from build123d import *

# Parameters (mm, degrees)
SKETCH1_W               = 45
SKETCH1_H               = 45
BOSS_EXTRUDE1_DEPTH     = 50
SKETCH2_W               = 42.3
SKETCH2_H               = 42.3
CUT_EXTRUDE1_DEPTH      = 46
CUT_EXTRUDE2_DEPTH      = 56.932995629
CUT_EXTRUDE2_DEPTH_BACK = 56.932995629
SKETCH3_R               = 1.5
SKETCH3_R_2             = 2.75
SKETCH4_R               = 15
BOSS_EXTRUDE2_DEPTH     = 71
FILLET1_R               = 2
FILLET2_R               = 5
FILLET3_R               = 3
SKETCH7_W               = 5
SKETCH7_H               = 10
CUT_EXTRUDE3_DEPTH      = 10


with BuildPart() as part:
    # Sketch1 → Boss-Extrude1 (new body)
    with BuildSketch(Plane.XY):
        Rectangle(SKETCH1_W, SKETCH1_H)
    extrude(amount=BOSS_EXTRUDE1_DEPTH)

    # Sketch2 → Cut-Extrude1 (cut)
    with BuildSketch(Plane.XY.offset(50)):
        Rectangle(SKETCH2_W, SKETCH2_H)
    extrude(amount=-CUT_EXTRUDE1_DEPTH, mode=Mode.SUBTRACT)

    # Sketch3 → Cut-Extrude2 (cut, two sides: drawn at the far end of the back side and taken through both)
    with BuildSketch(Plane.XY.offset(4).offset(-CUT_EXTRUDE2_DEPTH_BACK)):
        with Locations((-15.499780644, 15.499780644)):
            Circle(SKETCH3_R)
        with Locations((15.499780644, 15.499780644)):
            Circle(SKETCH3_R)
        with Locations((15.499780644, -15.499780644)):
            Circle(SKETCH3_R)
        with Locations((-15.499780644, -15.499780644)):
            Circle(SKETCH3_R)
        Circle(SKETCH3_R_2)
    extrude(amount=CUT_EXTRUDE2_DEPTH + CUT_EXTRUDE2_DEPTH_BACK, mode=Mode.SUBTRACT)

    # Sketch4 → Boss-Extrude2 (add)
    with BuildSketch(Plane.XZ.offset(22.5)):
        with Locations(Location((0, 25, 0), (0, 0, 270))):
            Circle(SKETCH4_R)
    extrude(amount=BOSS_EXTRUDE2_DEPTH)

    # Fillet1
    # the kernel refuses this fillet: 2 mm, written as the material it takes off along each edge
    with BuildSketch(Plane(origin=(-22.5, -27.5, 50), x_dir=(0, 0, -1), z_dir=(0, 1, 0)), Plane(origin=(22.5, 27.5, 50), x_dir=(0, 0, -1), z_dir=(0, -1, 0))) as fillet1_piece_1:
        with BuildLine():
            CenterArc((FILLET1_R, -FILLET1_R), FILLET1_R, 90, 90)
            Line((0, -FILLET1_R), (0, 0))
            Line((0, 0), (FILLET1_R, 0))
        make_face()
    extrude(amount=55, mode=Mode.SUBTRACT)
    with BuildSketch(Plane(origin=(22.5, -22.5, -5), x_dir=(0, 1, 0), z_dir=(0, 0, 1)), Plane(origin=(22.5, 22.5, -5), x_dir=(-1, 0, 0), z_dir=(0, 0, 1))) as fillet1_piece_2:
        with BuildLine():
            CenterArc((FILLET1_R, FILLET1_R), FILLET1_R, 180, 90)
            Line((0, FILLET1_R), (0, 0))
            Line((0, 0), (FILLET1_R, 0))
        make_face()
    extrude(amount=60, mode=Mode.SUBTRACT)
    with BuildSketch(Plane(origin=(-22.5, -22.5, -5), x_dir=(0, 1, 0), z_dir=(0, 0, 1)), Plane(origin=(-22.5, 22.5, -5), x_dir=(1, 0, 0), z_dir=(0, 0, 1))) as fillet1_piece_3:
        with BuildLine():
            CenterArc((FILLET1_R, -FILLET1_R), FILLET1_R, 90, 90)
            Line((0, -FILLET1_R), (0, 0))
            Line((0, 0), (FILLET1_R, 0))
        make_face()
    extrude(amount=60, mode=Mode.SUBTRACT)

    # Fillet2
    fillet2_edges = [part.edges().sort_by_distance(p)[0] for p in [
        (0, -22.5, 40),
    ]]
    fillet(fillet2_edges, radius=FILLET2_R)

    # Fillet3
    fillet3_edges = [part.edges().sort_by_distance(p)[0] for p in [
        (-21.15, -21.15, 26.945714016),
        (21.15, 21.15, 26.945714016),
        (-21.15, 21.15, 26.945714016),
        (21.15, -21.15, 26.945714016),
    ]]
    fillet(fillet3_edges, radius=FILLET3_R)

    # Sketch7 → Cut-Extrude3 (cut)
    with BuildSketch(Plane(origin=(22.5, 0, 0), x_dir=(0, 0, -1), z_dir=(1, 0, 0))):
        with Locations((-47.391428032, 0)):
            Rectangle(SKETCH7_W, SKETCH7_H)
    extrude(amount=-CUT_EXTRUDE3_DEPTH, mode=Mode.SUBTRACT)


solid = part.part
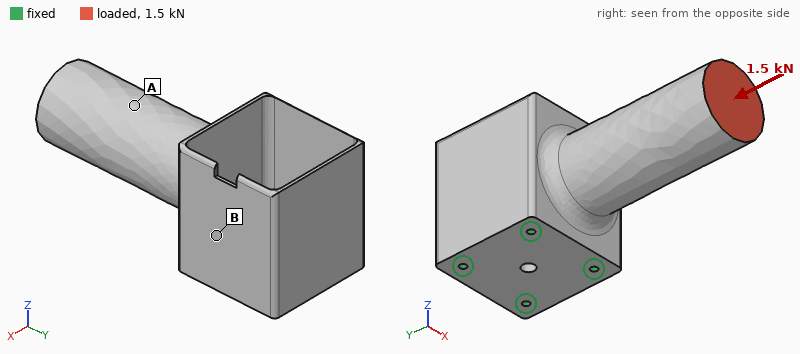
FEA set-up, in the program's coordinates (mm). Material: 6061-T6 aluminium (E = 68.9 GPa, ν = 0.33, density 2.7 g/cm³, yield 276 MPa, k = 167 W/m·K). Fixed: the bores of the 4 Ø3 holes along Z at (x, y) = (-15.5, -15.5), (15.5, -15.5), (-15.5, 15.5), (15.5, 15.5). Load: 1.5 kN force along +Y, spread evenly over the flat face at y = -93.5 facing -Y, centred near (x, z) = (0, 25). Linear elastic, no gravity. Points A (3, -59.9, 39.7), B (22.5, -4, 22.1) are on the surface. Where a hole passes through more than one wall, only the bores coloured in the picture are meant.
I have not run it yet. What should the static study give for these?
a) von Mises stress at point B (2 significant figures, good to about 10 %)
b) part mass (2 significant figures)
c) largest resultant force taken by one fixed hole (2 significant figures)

23 MPa
190 g
640 N
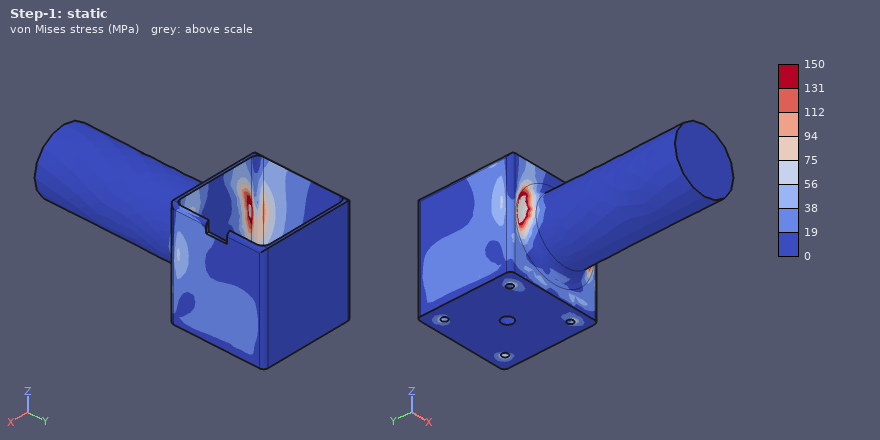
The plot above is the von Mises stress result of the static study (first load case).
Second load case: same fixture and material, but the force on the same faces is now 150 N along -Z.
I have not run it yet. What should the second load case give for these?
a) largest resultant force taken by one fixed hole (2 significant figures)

250 N
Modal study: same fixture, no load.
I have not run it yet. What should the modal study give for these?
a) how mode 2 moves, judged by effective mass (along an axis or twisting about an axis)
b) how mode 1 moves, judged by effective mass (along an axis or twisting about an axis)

along X
along Z
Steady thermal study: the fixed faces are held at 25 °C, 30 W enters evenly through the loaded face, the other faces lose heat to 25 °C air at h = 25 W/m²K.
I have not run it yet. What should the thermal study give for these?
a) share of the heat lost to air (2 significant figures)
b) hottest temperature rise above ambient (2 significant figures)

27 %
37 K
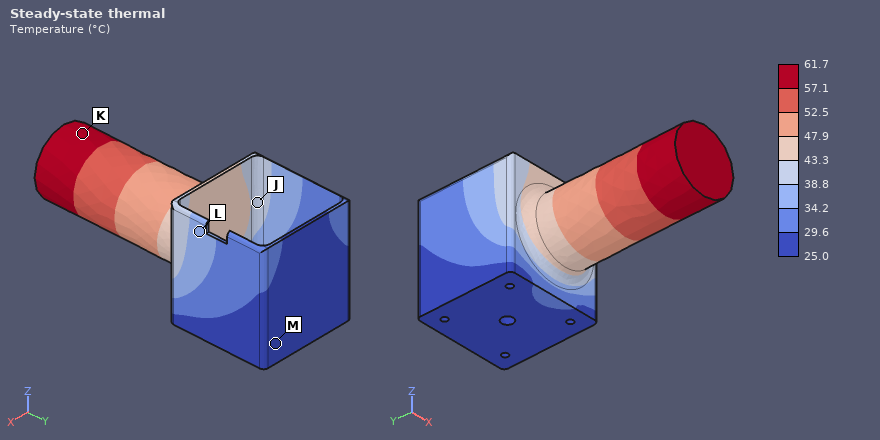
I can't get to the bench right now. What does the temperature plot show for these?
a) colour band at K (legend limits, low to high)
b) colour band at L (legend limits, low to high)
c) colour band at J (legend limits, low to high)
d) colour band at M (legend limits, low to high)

57.1 to 61.7 °C
34.2 to 38.8 °C
38.8 to 43.3 °C
25.0 to 29.6 °C
